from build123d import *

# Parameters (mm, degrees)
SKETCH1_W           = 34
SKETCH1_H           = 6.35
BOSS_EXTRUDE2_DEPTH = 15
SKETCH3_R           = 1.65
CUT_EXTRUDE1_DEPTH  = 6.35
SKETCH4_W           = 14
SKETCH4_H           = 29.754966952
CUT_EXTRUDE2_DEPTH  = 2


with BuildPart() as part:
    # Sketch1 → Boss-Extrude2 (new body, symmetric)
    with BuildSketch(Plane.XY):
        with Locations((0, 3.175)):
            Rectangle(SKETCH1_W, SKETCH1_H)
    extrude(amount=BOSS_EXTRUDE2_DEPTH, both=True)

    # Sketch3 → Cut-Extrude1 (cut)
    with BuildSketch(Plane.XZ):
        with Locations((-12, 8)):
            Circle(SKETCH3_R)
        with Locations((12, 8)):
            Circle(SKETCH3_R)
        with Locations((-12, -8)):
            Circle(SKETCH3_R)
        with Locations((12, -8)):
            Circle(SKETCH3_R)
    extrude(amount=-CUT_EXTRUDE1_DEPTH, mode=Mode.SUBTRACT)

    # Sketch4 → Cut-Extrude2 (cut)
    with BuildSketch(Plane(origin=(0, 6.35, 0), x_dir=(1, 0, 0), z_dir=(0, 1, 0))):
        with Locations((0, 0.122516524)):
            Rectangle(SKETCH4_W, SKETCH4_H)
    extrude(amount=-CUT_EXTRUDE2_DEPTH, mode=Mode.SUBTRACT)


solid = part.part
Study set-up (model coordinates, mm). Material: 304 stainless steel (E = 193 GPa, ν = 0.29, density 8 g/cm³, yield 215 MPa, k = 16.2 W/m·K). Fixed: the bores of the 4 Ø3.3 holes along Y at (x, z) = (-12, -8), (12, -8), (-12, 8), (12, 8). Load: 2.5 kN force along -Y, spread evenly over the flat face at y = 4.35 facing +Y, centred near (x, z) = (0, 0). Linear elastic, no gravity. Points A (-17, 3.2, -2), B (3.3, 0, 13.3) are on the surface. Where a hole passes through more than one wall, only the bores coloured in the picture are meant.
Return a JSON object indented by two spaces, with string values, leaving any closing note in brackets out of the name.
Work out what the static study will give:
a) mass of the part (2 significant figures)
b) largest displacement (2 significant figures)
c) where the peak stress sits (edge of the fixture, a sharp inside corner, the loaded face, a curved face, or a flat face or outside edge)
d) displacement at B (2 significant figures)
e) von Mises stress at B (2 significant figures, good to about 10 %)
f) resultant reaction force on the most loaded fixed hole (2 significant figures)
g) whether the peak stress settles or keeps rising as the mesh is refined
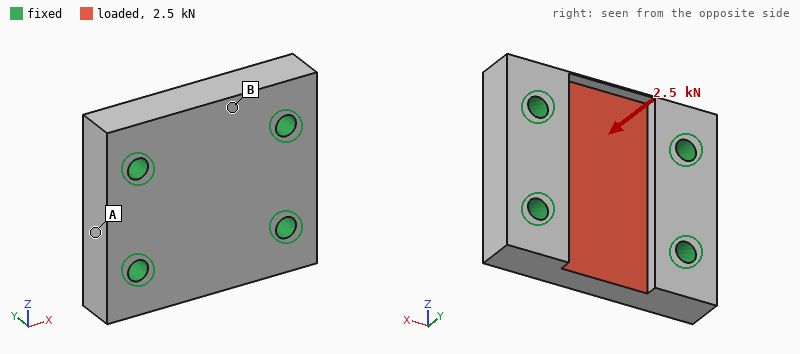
{
  "mass of the part": "43 g",
  "largest displacement": "3.5 µm",
  "where the peak stress sits": "edge of the fixture",
  "displacement at B": "2.6 µm",
  "von Mises stress at B": "22 MPa",
  "resultant reaction force on the most loaded fixed hole": "650 N",
  "whether the peak stress settles or keeps rising as the mesh is refined": "keeps rising"
}
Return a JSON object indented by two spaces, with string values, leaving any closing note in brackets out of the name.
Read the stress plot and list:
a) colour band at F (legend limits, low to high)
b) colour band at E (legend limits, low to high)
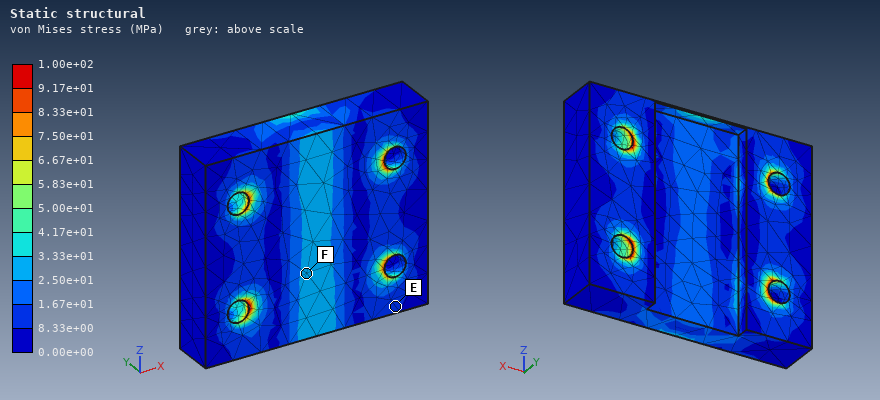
{
  "colour band at F": "2.50e+01 to 3.33e+01 MPa",
  "colour band at E": "8.33e+00 to 1.67e+01 MPa"
}
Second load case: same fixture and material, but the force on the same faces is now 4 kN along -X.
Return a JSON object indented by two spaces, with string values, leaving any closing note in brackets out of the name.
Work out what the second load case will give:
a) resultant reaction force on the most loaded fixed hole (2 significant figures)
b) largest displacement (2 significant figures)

{
  "resultant reaction force on the most loaded fixed hole": "1.0 kN",
  "largest displacement": "1.2 µm"
}
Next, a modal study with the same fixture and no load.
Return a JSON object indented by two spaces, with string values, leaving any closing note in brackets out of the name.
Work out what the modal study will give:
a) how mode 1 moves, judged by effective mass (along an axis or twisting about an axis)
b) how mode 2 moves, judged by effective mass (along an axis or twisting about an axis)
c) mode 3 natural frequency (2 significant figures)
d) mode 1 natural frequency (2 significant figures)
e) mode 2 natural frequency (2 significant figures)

{
  "how mode 1 moves, judged by effective mass": "along Y",
  "how mode 2 moves, judged by effective mass": "twisting about X",
  "mode 3 natural frequency": "50 kHz",
  "mode 1 natural frequency": "38 kHz",
  "mode 2 natural frequency": "42 kHz"
}
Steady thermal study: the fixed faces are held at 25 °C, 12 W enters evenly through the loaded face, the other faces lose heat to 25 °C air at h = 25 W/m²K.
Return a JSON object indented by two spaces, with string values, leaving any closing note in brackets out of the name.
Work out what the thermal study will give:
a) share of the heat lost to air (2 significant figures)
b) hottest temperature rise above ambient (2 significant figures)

{
  "share of the heat lost to air": "3.8 %",
  "hottest temperature rise above ambient": "24 K"
}
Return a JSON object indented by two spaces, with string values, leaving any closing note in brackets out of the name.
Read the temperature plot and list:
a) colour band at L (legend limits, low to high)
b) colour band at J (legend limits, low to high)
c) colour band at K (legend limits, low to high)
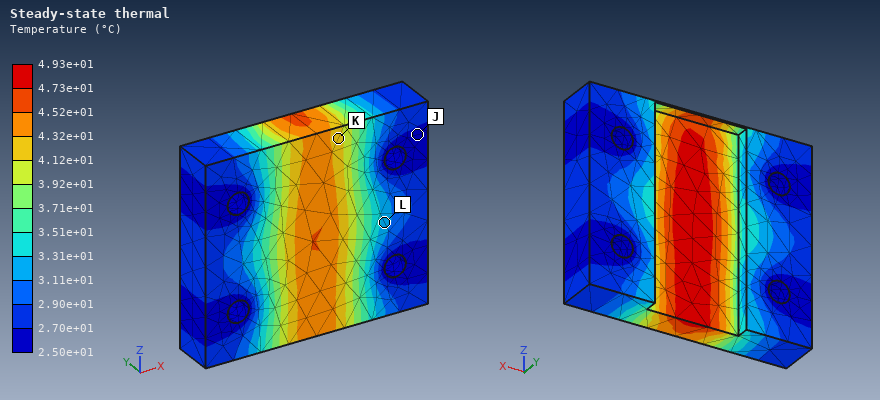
{
  "colour band at L": "3.11e+01 to 3.31e+01 °C",
  "colour band at J": "2.50e+01 to 2.70e+01 °C",
  "colour band at K": "4.12e+01 to 4.32e+01 °C"
}
